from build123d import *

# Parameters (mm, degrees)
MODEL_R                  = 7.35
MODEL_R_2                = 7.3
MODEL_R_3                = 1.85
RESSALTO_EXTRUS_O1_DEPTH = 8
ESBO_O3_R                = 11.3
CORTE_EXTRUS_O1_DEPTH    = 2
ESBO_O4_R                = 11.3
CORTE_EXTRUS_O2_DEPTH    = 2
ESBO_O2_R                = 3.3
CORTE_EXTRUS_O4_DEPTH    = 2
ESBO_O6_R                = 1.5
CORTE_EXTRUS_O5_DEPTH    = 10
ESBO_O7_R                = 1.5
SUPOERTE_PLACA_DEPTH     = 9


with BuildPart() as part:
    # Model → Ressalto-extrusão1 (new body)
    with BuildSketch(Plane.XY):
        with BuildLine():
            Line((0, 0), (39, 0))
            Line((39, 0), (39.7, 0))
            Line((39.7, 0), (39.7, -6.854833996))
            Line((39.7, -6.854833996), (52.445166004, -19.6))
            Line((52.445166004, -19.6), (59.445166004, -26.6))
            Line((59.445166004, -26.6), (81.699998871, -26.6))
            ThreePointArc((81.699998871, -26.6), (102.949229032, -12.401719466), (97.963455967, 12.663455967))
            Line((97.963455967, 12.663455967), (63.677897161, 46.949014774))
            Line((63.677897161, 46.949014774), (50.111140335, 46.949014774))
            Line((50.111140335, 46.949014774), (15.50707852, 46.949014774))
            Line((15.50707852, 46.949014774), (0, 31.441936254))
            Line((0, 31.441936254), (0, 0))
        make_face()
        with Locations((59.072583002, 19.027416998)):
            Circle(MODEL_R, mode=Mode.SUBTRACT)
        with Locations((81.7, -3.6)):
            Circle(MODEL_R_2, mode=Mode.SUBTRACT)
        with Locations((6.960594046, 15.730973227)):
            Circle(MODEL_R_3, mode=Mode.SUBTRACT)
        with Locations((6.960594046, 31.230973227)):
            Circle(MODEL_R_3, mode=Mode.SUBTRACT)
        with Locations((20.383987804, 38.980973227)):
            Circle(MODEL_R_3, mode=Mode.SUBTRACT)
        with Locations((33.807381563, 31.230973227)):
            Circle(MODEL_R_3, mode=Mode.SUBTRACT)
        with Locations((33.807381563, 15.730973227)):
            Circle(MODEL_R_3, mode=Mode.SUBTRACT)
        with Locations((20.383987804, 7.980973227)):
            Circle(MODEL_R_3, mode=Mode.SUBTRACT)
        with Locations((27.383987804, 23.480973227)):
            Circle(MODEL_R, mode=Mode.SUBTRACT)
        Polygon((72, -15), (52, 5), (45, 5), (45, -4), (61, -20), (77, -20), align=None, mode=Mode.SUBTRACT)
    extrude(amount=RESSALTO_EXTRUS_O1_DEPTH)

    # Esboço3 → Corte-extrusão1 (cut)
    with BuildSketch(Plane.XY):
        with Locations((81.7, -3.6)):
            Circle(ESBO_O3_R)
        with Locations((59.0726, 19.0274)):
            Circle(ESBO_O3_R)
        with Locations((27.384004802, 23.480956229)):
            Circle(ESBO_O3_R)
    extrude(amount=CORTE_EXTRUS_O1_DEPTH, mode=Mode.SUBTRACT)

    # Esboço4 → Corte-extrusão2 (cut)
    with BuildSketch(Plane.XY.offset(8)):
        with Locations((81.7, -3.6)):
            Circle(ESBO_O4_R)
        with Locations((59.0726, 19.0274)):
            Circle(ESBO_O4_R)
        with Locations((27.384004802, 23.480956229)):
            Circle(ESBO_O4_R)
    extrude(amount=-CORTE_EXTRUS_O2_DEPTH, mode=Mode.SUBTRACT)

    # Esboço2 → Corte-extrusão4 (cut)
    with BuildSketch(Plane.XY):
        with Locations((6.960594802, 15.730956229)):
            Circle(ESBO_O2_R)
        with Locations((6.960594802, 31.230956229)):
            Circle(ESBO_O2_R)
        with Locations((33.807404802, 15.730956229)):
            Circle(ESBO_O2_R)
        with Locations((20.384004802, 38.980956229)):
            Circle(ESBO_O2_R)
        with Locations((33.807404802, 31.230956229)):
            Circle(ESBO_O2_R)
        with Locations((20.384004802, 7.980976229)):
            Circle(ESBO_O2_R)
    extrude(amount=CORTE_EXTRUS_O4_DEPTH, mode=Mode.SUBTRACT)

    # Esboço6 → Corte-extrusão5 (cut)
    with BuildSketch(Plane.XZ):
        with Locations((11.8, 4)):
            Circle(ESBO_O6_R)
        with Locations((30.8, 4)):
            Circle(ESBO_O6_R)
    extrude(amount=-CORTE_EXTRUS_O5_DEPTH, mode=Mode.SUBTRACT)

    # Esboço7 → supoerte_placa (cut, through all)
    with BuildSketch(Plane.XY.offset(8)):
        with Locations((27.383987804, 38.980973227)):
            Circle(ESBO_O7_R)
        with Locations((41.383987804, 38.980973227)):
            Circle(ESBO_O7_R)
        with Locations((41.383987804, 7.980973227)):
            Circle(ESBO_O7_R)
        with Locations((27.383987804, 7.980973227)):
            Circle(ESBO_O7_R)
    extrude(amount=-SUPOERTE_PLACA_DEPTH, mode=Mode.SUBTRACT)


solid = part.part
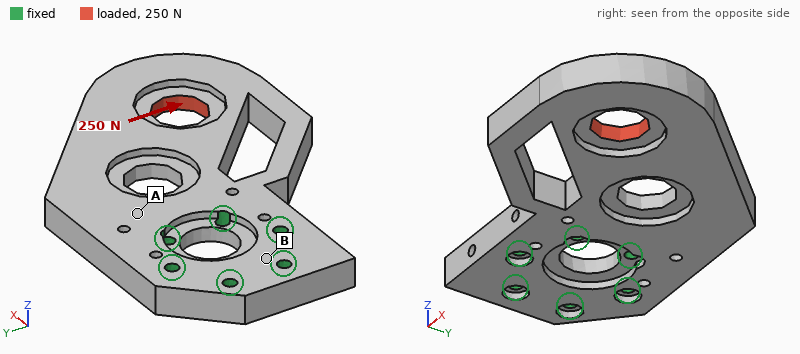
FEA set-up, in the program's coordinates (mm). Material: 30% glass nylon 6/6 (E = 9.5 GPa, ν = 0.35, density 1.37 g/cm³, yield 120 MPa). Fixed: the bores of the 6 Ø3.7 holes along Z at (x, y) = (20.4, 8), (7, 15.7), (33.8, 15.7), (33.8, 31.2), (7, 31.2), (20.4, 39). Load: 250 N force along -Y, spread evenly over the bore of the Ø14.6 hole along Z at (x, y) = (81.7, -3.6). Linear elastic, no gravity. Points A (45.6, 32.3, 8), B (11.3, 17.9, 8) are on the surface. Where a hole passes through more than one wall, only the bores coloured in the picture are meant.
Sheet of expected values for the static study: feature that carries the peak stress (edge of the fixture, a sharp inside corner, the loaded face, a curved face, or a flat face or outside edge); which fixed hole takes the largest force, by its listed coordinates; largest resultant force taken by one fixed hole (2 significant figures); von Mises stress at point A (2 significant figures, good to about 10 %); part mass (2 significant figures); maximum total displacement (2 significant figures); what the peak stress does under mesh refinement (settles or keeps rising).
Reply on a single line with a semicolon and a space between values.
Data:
edge of the fixture; (33.8, 15.7); 280 N; 1.7 MPa; 44 g; 91 µm; keeps rising
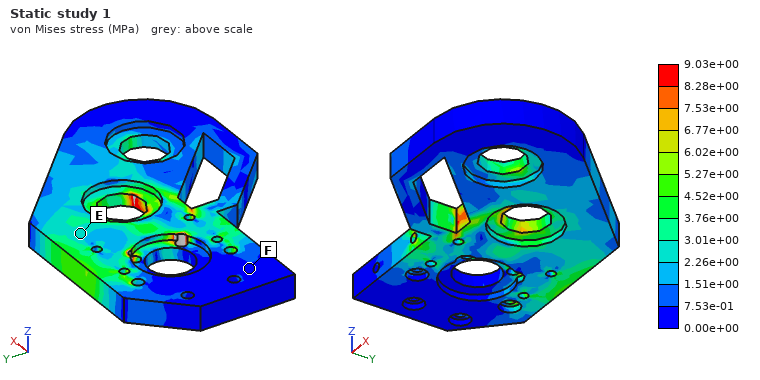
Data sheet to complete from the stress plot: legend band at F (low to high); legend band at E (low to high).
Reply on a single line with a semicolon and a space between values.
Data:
0.00e+00 to 7.53e-01 MPa; 2.26e+00 to 3.01e+00 MPa
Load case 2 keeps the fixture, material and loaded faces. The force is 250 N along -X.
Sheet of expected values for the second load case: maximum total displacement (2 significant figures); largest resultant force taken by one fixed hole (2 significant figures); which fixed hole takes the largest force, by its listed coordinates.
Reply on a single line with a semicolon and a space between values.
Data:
63 µm; 220 N; (33.8, 15.7)
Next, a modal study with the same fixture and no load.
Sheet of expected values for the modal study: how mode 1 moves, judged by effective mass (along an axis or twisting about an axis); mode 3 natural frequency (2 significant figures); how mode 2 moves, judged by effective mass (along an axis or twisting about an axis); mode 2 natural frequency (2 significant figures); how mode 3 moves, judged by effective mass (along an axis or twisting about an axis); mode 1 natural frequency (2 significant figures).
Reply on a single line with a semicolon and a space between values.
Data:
along Z; 2000 Hz; twisting about X; 1400 Hz; along Y; 520 Hz
